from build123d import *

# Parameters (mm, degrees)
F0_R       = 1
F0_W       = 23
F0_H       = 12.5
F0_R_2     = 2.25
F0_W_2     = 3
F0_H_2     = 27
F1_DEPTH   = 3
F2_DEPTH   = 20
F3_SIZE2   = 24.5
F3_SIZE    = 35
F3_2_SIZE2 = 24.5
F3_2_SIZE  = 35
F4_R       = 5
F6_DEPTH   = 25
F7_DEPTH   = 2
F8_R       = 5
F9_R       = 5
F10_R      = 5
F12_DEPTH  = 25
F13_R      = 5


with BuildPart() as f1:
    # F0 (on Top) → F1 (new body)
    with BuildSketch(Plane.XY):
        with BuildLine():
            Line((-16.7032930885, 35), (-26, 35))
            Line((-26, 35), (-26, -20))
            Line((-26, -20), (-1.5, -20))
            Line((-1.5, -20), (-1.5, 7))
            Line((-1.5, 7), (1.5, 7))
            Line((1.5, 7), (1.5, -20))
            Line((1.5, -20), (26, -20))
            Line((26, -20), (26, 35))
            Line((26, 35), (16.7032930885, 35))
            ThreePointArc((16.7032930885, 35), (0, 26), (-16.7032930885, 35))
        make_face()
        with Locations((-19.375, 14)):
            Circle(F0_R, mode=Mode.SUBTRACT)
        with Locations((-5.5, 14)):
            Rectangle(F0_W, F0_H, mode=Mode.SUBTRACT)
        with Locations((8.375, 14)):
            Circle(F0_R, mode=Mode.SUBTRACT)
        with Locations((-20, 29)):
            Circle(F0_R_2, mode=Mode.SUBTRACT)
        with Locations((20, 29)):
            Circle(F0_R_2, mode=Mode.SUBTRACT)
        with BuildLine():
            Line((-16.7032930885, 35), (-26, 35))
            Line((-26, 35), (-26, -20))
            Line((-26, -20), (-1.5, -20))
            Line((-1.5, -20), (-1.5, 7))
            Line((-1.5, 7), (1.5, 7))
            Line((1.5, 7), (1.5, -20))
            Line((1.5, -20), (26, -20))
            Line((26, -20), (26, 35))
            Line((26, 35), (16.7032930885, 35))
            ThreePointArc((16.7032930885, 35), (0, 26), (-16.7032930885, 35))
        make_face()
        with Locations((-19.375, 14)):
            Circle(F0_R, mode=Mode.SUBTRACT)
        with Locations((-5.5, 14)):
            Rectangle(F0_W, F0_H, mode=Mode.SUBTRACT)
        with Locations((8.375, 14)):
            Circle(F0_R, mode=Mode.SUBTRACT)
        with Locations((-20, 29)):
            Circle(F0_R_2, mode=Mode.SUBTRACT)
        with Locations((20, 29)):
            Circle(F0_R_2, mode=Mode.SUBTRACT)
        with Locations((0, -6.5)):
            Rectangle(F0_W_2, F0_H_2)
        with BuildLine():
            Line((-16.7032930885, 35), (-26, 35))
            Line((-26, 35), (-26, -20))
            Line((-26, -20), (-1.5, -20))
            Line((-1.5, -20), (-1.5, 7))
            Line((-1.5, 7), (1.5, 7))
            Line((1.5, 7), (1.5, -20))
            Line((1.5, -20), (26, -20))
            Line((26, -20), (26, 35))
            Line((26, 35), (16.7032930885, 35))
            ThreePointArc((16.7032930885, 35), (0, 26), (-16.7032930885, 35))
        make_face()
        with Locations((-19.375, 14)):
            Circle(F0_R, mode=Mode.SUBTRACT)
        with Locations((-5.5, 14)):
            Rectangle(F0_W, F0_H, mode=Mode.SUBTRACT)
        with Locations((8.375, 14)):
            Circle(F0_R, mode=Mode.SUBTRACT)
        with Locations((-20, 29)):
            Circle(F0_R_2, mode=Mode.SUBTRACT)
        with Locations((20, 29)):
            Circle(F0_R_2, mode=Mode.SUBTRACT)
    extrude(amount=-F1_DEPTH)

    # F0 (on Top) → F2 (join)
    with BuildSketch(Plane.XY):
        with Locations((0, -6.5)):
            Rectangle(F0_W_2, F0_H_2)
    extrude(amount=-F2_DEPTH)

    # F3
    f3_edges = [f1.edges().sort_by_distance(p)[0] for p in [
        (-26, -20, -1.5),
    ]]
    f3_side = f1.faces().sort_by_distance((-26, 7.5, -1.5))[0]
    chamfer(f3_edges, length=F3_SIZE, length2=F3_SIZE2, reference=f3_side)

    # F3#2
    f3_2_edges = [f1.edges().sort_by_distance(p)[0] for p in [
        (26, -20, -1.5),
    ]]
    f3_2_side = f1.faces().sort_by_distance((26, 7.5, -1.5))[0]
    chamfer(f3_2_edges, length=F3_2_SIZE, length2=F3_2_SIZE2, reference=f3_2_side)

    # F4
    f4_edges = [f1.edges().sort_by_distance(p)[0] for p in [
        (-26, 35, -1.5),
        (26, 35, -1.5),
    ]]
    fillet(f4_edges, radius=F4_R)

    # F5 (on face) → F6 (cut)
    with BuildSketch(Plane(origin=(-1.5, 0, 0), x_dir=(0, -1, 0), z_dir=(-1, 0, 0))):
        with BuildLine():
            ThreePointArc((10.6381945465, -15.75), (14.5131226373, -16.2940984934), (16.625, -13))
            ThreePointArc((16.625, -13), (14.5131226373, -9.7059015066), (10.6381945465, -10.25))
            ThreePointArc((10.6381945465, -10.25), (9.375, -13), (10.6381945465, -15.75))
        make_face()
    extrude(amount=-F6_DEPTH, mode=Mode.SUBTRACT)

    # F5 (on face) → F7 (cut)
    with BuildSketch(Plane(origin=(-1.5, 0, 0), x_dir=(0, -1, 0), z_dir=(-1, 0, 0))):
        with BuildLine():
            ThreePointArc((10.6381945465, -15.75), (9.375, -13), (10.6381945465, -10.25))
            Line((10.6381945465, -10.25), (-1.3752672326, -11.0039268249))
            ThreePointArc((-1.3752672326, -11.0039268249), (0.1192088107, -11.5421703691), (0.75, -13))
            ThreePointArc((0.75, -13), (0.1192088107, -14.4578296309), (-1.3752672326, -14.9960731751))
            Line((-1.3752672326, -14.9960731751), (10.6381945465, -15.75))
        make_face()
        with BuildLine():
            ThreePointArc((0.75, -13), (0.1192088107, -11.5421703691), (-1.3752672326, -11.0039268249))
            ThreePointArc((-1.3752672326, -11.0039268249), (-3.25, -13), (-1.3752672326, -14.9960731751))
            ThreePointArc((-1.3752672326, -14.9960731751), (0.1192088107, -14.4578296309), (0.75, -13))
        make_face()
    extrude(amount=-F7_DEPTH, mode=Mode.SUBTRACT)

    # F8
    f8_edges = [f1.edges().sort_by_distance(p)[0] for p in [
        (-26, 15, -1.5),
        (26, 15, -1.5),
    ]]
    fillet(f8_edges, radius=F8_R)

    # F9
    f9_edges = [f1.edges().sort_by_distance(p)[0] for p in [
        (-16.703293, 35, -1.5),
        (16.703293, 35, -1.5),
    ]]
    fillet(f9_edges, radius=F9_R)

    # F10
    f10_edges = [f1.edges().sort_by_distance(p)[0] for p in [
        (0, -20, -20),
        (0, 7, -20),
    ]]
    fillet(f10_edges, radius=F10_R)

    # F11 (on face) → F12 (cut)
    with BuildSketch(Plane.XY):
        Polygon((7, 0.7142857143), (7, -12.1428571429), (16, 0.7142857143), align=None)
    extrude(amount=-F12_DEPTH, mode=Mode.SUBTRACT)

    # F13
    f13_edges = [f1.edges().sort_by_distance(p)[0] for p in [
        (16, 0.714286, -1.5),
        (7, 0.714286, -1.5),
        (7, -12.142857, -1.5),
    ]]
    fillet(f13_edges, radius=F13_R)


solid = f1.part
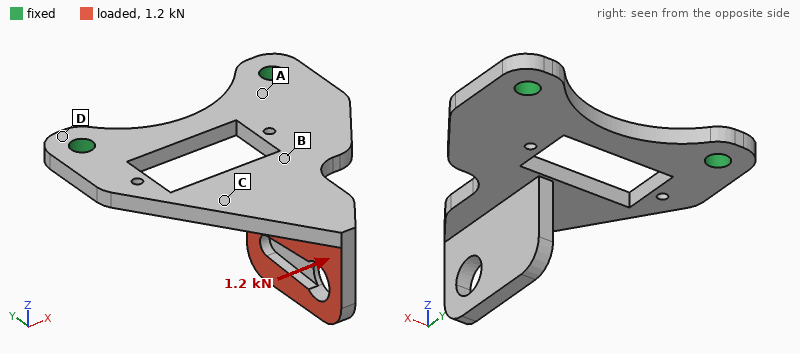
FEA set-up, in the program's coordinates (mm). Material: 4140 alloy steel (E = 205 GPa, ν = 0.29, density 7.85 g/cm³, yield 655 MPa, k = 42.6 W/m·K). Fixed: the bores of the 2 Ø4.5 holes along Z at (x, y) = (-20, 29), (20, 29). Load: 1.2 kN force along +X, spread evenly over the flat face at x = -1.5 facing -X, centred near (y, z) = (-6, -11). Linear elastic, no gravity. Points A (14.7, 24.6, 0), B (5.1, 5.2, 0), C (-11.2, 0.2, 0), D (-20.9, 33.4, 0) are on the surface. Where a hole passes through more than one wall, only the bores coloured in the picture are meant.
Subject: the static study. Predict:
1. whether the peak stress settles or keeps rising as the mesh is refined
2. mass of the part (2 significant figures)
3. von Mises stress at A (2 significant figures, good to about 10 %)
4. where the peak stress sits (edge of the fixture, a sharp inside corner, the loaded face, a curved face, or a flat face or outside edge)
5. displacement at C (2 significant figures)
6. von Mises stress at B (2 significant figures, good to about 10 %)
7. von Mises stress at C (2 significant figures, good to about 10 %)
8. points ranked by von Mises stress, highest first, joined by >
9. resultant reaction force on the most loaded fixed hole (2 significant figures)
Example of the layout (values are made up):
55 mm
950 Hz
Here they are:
keeps rising
42 g
95 MPa
a sharp inside corner
0.13 mm
260 MPa
180 MPa
B > C > A > D
1.1 kN
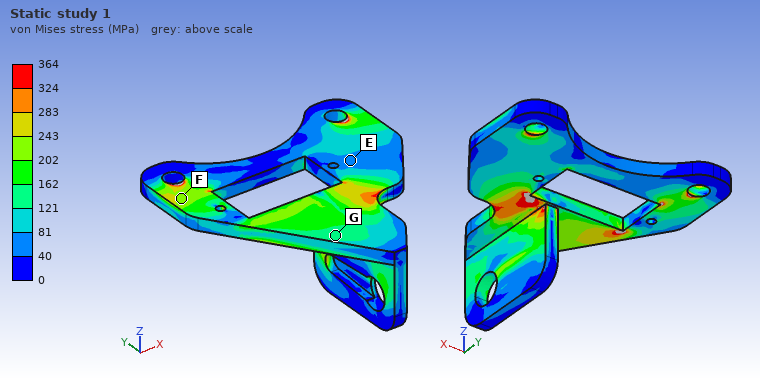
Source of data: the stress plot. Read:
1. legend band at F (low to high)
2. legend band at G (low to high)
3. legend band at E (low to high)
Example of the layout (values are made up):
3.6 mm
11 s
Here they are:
202 to 243 MPa
121 to 162 MPa
40 to 81 MPa
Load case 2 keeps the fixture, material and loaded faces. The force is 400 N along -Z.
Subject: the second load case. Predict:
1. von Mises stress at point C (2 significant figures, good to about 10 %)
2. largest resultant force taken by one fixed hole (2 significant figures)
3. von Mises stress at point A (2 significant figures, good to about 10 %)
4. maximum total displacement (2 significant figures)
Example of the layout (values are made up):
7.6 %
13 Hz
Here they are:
83 MPa
210 N
240 MPa
0.90 mm
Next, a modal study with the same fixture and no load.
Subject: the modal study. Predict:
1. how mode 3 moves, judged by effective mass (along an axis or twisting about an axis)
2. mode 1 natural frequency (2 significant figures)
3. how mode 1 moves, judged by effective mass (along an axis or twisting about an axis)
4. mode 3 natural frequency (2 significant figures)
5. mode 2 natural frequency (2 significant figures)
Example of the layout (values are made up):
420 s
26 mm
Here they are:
along Z
940 Hz
along Z
4000 Hz
3300 Hz
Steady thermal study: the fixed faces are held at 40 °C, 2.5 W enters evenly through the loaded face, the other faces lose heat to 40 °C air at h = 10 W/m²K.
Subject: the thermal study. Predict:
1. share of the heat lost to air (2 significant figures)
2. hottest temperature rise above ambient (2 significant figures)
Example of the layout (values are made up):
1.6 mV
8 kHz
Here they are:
26 %
36 K
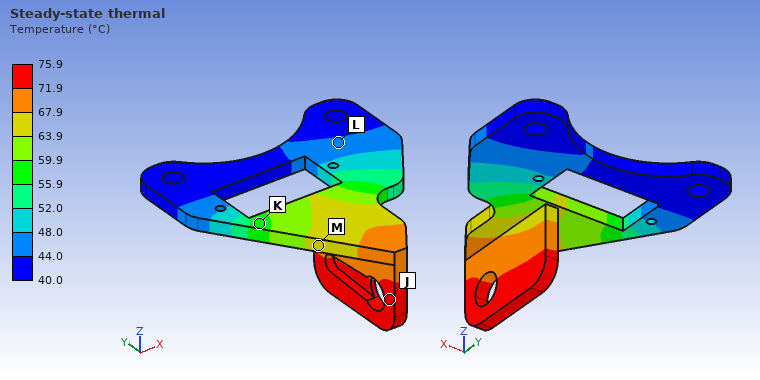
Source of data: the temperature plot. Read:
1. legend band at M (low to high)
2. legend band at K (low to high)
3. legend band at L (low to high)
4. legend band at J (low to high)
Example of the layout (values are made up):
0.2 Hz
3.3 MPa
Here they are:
63.9 to 67.9 °C
55.9 to 59.9 °C
44.0 to 48.0 °C
71.9 to 75.9 °C
